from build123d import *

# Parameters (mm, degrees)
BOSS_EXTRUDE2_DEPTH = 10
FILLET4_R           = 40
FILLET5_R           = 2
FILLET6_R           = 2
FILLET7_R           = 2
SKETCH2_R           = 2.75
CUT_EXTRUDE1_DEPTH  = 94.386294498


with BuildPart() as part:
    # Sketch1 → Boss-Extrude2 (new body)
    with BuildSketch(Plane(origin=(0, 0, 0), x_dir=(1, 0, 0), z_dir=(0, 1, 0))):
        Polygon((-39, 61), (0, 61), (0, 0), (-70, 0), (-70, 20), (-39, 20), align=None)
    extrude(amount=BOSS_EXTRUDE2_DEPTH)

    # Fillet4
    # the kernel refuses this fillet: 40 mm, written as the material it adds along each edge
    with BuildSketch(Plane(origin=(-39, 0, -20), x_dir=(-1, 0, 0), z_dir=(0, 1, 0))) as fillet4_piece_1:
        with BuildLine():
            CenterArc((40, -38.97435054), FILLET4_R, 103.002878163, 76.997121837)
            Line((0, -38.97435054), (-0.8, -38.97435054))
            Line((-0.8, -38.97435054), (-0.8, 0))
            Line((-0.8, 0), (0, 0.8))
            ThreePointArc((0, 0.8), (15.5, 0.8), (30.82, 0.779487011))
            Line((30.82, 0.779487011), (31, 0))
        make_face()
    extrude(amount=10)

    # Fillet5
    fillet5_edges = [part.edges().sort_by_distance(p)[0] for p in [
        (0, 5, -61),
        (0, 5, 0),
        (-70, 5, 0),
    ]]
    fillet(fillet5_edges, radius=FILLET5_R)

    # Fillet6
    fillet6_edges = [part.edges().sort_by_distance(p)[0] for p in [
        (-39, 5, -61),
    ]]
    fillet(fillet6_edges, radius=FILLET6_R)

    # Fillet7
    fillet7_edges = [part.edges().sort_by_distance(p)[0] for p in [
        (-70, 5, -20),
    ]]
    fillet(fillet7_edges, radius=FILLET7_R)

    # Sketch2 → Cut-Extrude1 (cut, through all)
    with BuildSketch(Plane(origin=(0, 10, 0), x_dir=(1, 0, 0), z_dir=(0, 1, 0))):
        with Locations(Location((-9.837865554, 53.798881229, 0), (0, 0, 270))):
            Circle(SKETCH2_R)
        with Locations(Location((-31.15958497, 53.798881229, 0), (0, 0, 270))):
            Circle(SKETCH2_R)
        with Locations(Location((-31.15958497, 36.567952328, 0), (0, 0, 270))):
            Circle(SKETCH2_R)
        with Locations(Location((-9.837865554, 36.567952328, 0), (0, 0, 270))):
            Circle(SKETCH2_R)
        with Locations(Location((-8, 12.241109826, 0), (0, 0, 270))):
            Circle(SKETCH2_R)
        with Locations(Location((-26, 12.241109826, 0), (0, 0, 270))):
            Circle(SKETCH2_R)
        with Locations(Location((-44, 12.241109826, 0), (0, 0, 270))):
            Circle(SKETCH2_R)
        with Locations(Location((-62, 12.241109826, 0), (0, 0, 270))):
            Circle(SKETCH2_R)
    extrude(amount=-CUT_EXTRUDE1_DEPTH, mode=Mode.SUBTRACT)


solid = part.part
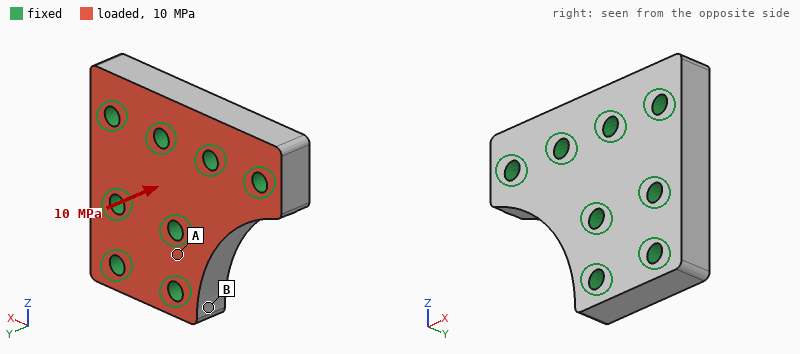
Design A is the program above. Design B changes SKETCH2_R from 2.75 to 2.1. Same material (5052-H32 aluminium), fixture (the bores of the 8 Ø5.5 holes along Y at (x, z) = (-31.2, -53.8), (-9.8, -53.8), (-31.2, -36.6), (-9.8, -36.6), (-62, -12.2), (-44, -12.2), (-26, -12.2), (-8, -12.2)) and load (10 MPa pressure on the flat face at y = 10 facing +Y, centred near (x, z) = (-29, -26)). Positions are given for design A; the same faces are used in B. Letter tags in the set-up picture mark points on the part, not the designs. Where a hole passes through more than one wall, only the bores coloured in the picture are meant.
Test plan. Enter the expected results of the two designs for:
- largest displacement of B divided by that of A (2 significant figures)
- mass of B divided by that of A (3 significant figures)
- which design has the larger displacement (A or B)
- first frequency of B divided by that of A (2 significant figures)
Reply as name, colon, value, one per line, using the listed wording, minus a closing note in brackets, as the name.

largest displacement of B divided by that of A: 1.1
mass of B divided by that of A: 1.03
which design has the larger displacement: B
first frequency of B divided by that of A: 0.91
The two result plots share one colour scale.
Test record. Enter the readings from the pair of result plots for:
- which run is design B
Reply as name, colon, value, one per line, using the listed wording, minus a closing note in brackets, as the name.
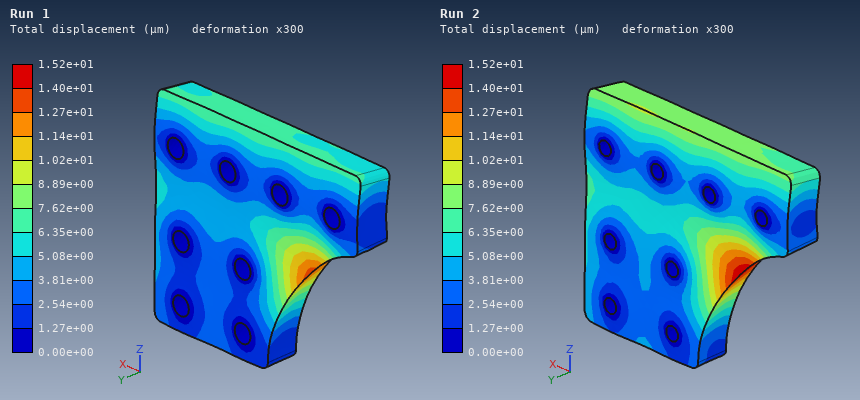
which run is design B: Run 2
